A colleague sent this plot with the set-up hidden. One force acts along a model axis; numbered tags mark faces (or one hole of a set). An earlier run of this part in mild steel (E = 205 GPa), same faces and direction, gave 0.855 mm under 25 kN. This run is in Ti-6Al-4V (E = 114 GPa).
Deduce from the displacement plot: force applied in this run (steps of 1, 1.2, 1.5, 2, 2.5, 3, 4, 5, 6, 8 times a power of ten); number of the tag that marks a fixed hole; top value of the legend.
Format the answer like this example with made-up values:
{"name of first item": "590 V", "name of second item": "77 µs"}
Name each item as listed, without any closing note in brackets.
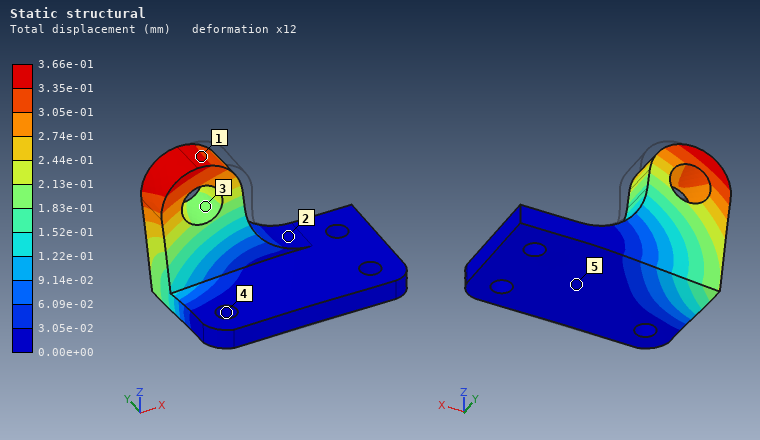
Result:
{"force applied in this run": "6 kN", "number of the tag that marks a fixed hole": "4", "top value of the legend": "3.66e-01 mm"}
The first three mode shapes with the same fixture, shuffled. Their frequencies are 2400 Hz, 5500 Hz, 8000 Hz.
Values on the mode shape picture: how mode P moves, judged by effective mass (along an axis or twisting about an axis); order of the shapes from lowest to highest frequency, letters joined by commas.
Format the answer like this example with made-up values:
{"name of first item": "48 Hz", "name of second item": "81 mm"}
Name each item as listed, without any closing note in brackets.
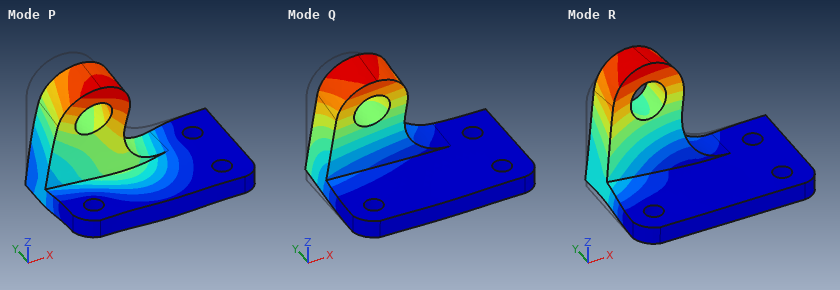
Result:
{"how mode P moves, judged by effective mass": "along Z", "order of the shapes from lowest to highest frequency, letters joined by commas": "Q, R, P"}
